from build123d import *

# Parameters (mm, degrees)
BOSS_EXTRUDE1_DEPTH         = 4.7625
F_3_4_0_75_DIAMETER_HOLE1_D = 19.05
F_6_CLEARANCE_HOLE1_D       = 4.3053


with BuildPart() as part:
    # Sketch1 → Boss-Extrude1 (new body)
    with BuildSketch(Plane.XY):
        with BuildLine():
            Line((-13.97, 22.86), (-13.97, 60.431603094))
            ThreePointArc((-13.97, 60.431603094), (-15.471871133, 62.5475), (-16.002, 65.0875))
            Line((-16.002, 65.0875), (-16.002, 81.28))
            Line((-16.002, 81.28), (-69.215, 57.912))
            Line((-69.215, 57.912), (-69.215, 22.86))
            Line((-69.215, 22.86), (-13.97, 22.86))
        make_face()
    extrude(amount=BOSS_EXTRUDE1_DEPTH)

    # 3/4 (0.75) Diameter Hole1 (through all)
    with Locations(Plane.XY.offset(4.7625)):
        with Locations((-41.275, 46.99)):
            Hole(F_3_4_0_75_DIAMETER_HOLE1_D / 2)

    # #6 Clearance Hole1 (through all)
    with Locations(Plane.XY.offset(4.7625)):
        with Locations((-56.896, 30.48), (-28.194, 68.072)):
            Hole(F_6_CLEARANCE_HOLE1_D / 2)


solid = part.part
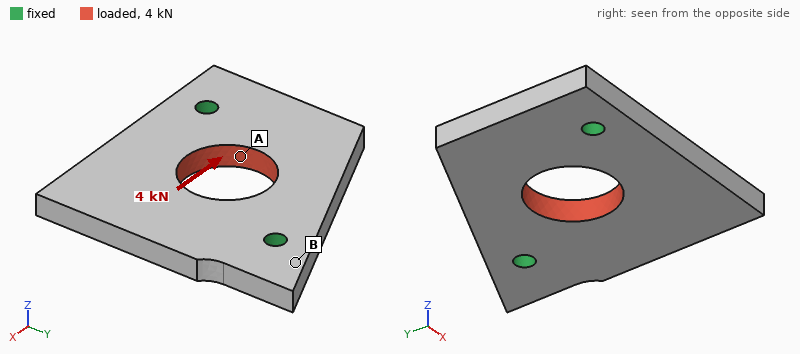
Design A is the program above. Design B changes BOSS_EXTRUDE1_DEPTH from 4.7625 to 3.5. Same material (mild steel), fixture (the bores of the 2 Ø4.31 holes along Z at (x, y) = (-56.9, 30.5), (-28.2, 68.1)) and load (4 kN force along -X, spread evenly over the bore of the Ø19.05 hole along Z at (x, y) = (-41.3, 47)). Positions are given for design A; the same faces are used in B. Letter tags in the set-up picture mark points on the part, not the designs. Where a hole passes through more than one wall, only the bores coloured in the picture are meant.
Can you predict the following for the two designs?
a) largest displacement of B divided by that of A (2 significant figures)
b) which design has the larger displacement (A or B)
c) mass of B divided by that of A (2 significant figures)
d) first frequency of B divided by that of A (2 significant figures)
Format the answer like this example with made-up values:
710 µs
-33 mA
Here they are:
1.4
B
0.73
0.76
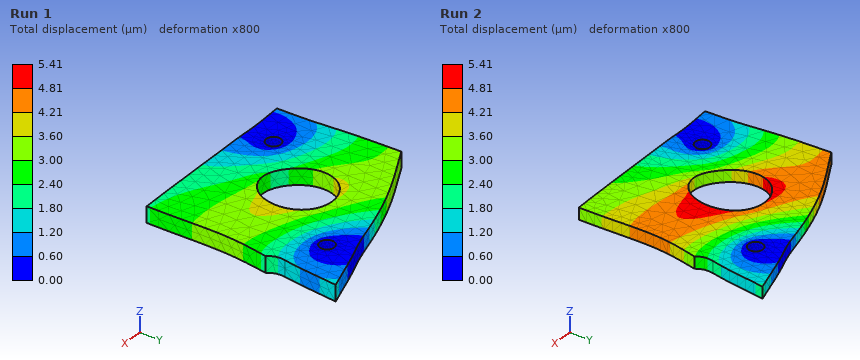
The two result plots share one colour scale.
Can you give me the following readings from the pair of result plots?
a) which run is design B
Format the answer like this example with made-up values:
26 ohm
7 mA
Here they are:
Run 2
